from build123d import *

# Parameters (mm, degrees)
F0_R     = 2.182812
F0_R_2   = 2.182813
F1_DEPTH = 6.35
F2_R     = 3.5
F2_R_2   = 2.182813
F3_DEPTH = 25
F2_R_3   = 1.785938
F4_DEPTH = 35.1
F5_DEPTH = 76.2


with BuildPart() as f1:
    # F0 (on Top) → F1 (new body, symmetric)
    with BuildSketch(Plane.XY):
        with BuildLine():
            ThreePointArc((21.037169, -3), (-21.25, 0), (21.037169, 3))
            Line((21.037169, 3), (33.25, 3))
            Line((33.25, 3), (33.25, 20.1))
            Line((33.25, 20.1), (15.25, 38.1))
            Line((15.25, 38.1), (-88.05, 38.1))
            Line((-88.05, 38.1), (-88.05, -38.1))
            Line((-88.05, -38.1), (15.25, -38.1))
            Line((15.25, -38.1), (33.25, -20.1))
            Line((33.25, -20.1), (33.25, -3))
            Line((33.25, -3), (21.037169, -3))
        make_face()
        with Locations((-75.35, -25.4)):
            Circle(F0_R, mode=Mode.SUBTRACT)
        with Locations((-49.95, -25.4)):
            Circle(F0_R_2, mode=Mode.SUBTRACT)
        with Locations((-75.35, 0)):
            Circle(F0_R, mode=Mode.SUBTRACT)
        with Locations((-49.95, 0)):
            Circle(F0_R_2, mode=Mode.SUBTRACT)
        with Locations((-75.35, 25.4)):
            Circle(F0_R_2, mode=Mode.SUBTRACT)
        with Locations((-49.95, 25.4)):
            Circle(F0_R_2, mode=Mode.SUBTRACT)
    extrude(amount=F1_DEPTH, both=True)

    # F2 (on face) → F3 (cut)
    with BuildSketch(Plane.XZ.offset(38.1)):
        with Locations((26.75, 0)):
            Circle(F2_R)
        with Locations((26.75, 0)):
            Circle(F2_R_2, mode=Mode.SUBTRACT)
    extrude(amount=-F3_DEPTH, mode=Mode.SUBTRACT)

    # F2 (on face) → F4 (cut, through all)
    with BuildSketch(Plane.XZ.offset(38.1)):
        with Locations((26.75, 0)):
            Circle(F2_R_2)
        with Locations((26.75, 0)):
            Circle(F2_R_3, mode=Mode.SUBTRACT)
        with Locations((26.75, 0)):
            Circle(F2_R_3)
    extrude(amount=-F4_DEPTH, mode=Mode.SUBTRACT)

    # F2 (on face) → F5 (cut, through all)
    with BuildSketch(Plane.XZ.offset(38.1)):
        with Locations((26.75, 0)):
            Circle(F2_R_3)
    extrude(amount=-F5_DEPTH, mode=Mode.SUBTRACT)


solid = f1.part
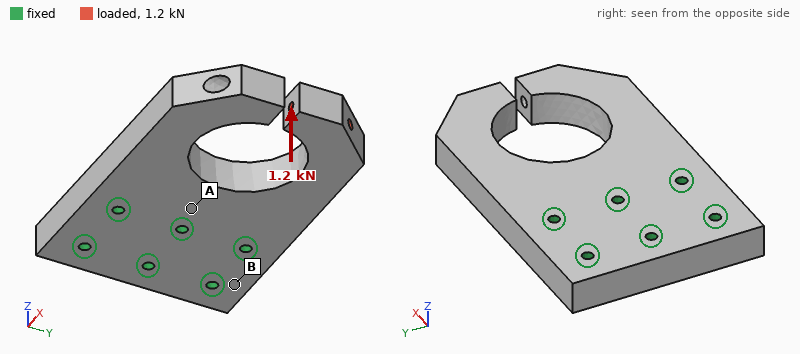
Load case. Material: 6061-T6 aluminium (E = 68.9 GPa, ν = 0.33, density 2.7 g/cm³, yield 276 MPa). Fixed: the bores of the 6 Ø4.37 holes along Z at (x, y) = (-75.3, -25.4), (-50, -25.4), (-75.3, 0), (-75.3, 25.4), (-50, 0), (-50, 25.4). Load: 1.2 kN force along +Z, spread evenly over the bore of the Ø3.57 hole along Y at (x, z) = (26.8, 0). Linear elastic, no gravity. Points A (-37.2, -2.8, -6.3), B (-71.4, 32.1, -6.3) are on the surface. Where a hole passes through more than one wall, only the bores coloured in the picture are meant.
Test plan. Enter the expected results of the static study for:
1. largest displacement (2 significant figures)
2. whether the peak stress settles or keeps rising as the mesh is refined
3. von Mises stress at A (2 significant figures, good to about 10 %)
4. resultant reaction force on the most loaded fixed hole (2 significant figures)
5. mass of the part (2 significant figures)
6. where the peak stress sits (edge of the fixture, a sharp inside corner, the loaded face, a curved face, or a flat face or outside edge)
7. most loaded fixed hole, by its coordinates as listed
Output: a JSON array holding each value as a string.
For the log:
["0.68 mm", "keeps rising", "36 MPa", "1.3 kN", "250 g", "edge of the fixture", "(-50, 0)"]
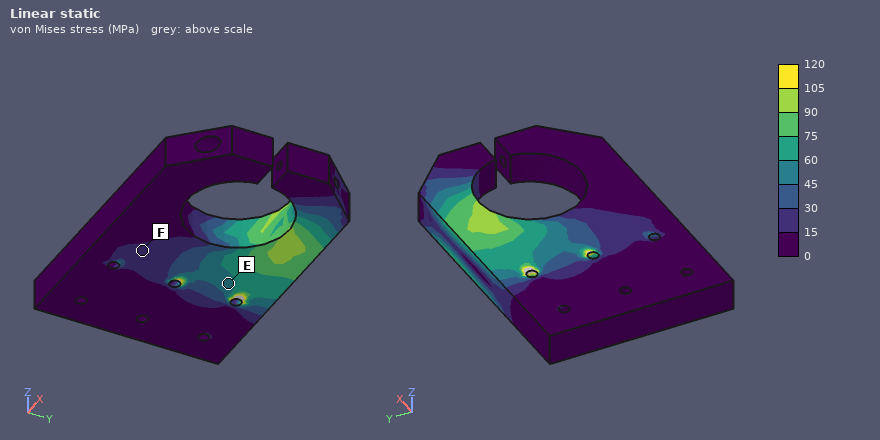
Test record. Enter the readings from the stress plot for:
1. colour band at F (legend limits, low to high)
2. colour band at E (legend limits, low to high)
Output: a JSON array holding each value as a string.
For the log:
["15 to 30 MPa", "45 to 60 MPa"]
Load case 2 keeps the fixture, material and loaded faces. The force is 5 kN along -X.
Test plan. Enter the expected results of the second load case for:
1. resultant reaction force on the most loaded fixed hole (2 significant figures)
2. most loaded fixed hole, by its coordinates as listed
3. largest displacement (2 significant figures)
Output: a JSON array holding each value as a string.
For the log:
["2.6 kN", "(-50, 25.4)", "0.31 mm"]
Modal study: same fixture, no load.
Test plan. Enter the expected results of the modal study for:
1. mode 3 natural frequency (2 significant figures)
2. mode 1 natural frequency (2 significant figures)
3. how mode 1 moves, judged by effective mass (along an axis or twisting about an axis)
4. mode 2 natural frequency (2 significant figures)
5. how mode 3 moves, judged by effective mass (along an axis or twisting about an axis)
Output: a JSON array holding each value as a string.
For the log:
["3700 Hz", "1700 Hz", "along Z", "1900 Hz", "along Y"]
